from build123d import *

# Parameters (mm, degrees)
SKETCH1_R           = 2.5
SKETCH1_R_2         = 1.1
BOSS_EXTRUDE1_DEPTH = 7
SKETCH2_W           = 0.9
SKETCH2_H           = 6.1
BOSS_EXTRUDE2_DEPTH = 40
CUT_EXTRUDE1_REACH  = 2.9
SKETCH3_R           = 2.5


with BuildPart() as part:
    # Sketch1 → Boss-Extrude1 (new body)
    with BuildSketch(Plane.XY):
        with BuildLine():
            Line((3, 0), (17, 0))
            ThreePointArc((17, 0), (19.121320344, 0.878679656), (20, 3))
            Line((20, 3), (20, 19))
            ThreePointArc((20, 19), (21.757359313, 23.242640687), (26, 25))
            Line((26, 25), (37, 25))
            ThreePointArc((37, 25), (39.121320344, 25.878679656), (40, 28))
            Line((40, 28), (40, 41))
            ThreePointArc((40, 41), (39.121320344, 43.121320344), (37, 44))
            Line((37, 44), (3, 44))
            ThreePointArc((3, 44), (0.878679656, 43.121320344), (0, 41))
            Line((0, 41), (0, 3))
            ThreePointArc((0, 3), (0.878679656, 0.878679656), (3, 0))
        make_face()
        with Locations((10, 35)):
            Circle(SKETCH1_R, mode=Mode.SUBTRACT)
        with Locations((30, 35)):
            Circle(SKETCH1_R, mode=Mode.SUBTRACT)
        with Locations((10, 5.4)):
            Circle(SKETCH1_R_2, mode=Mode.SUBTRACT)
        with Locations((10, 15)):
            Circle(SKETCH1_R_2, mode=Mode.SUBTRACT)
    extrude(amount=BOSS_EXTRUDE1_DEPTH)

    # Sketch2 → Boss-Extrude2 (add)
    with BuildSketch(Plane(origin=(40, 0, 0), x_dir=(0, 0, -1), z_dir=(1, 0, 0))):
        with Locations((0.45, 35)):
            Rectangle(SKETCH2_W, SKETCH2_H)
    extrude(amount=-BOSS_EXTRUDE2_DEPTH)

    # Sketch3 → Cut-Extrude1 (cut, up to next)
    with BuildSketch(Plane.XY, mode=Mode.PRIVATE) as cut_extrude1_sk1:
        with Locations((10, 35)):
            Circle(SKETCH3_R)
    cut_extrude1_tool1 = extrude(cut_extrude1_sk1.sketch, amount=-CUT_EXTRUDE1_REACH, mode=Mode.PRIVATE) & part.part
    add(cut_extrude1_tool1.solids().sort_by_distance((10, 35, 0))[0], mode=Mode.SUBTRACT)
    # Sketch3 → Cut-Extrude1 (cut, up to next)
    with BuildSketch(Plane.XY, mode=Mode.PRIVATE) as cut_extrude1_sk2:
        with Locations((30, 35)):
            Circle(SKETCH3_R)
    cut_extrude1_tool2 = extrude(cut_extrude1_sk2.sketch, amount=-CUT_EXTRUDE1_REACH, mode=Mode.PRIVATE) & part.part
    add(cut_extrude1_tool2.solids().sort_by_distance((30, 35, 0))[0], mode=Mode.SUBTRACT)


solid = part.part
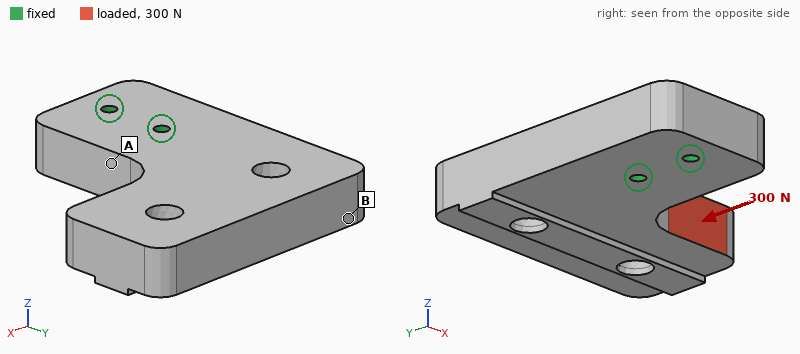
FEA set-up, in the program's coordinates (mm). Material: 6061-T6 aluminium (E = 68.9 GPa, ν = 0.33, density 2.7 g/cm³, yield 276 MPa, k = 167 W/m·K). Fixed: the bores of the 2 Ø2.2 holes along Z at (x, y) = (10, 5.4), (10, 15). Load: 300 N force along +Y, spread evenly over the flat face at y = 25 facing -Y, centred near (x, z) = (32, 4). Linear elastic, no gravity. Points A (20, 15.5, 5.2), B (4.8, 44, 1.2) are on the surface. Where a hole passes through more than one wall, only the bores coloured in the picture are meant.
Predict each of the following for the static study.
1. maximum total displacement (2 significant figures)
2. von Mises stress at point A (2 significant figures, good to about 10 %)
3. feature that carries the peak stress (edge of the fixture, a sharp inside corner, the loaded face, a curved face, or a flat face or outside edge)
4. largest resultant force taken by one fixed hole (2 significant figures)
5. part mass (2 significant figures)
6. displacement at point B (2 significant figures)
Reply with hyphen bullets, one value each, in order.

- 26 µm
- 15 MPa
- edge of the fixture
- 590 N
- 23 g
- 16 µm
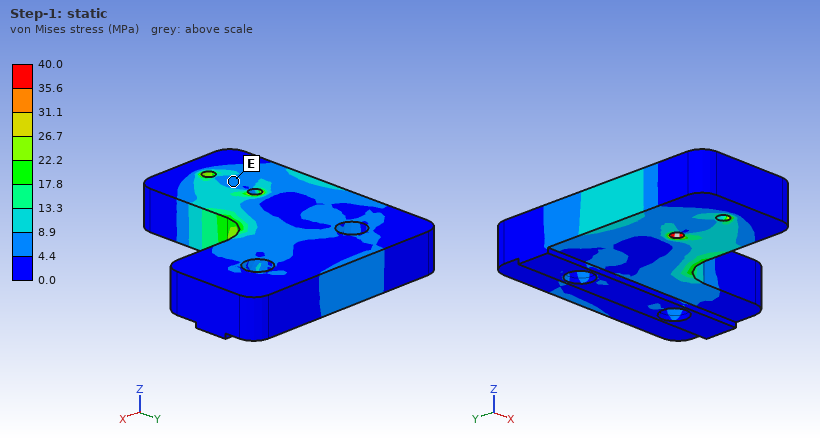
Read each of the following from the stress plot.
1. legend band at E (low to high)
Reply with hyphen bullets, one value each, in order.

- 4.4 to 8.9 MPa
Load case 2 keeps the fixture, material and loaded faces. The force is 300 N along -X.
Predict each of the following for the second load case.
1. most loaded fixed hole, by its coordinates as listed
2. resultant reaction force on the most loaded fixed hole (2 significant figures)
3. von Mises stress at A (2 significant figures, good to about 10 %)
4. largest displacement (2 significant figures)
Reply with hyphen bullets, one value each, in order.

- (10, 15)
- 550 N
- 7.3 MPa
- 7.2 µm
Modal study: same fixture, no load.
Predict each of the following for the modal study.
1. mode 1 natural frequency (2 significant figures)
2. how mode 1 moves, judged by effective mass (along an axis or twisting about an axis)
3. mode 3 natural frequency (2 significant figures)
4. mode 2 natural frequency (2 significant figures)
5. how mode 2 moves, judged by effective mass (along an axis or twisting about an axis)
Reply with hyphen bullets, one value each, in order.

- 3400 Hz
- along Z
- 6500 Hz
- 5700 Hz
- along X
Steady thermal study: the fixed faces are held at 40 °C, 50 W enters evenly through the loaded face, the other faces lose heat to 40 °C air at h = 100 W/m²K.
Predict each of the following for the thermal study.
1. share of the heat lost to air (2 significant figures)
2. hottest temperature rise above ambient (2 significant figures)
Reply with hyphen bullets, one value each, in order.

- 21 %
- 78 K
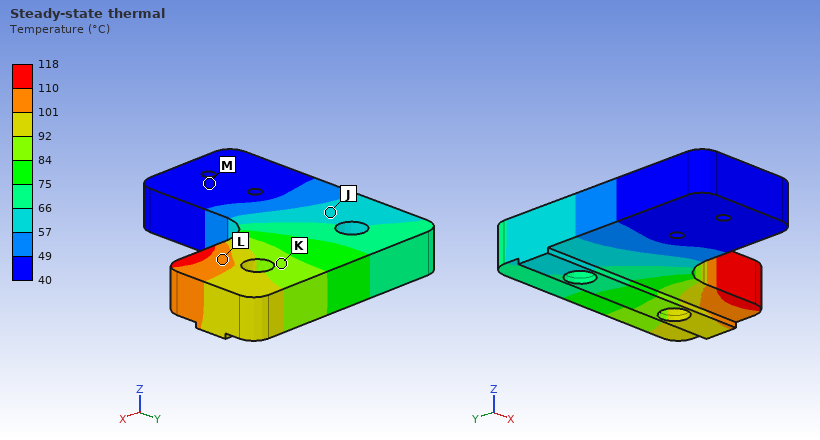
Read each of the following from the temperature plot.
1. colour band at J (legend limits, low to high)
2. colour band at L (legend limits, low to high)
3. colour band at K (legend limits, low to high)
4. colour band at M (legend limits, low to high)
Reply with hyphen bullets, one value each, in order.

- 57 to 66 °C
- 101 to 110 °C
- 84 to 92 °C
- 40 to 49 °C
